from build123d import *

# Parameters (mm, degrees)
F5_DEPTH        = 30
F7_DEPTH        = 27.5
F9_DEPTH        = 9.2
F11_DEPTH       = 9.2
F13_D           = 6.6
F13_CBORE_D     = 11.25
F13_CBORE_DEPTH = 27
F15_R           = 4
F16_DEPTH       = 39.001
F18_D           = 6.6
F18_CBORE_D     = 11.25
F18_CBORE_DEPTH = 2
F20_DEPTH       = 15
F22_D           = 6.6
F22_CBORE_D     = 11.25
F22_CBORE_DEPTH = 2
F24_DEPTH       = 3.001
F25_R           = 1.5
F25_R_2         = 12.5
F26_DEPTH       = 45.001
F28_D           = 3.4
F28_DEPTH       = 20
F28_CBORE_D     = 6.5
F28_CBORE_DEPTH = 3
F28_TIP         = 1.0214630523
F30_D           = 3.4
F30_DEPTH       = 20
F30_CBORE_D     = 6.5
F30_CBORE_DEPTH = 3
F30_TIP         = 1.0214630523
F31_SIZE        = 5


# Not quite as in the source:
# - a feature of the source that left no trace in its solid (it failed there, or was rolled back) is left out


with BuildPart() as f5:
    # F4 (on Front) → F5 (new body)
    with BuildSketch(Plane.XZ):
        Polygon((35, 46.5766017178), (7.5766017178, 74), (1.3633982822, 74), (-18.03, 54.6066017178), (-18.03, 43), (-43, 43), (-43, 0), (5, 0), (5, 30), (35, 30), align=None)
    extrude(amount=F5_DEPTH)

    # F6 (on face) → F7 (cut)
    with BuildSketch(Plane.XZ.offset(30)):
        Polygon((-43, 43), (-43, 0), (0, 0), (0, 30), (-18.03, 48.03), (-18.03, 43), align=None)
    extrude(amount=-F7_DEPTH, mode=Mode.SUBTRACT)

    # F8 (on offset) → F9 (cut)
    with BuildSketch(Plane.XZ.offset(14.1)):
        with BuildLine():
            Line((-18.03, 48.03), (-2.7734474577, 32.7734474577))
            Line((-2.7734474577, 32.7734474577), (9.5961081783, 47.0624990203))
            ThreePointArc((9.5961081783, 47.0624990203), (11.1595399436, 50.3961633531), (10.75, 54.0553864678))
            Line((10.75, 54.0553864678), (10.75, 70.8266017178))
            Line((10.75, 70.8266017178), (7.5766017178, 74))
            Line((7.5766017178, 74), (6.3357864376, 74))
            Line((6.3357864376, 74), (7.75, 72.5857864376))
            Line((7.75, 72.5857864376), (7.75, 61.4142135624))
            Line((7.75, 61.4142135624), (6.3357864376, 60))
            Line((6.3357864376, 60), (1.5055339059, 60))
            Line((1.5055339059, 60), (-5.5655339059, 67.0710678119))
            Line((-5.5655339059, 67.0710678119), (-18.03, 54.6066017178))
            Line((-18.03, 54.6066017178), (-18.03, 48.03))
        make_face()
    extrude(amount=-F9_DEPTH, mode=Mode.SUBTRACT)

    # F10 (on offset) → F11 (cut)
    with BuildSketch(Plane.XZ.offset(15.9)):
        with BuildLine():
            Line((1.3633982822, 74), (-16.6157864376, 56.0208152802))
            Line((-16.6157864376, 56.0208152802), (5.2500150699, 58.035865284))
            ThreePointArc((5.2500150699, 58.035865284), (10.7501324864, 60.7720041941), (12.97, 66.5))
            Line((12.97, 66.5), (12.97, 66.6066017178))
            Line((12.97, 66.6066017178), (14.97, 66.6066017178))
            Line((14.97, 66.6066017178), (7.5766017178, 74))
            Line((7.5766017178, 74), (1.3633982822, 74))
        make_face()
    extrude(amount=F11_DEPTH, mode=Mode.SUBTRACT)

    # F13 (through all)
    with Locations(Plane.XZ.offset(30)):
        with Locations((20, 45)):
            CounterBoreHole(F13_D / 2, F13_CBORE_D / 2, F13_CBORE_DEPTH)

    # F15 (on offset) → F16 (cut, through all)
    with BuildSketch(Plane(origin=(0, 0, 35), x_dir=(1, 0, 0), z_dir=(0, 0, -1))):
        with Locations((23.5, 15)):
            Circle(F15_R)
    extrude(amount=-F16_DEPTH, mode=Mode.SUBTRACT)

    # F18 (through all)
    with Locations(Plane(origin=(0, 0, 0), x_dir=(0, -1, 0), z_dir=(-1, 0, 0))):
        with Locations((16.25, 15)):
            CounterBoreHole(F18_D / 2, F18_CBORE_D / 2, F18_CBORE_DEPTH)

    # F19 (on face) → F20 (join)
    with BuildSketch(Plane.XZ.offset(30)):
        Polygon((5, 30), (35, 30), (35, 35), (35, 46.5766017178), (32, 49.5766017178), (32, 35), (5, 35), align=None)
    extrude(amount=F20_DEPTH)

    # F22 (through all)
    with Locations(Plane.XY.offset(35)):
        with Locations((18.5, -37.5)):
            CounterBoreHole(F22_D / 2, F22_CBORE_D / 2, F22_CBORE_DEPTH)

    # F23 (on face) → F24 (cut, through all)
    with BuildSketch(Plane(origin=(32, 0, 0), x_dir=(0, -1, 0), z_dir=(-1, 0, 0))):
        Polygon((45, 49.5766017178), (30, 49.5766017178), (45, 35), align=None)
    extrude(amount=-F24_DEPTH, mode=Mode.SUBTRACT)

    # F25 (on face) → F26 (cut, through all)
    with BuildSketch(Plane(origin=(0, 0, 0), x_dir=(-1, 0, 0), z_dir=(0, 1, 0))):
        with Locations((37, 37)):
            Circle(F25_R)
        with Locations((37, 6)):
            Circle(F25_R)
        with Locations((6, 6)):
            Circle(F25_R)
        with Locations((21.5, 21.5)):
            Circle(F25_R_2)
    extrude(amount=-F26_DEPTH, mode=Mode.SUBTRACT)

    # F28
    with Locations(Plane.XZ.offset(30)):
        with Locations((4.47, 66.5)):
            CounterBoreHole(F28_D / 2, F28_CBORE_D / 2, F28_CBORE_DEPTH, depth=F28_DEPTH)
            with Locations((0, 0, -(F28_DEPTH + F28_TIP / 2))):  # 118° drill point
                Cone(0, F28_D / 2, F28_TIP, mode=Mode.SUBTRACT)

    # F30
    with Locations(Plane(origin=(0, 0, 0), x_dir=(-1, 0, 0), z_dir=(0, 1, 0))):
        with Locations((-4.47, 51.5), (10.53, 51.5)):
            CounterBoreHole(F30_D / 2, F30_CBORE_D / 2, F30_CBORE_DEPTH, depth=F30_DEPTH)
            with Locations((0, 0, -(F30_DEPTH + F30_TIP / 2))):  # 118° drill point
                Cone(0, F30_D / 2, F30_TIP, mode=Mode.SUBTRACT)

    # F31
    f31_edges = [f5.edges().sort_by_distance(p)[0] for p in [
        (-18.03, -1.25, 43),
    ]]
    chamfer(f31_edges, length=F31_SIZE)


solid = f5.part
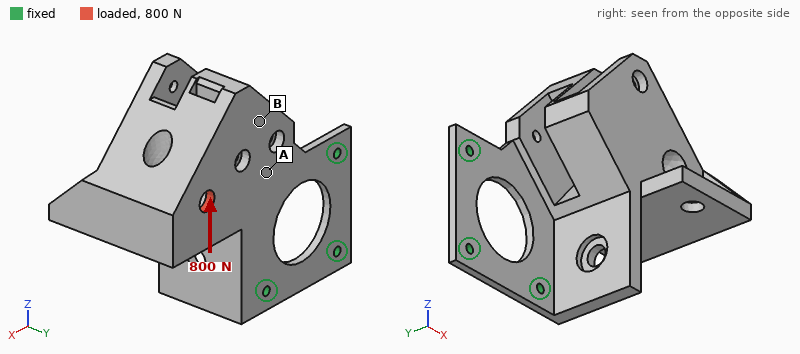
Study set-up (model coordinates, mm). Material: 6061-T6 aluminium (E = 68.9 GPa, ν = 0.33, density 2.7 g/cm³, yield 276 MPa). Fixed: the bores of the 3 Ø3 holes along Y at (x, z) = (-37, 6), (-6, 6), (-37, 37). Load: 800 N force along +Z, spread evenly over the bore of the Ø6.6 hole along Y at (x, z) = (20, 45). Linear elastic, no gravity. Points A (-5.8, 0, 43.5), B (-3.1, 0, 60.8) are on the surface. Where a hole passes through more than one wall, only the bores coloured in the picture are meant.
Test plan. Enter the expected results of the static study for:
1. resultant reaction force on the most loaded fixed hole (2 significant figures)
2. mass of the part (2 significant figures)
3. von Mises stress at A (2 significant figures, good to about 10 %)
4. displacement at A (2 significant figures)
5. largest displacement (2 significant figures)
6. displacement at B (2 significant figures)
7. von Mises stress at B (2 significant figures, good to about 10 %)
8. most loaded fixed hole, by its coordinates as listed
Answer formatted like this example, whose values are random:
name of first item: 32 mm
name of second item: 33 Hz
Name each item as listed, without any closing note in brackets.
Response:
resultant reaction force on the most loaded fixed hole: 1.1 kN
mass of the part: 120 g
von Mises stress at A: 13 MPa
displacement at A: 13 µm
largest displacement: 55 µm
displacement at B: 34 µm
von Mises stress at B: 4.9 MPa
most loaded fixed hole, by its coordinates as listed: (-6, 6)
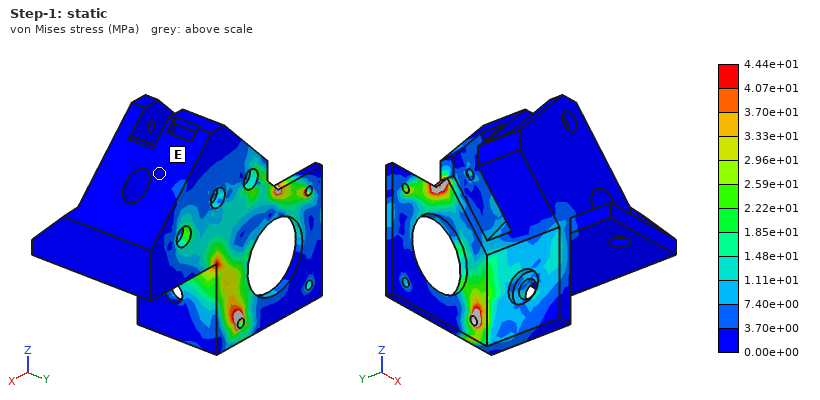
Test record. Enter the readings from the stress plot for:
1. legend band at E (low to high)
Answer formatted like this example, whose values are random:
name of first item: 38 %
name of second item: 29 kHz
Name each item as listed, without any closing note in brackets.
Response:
legend band at E: 0.00e+00 to 3.70e+00 MPa
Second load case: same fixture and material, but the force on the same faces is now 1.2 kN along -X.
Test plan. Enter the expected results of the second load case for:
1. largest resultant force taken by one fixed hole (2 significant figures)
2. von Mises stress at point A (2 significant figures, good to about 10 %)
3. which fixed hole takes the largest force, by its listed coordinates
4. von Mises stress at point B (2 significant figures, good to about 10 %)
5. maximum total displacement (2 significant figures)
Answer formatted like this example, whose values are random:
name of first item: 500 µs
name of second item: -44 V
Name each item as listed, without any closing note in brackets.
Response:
largest resultant force taken by one fixed hole: 1.2 kN
von Mises stress at point A: 26 MPa
which fixed hole takes the largest force, by its listed coordinates: (-37, 37)
von Mises stress at point B: 8.1 MPa
maximum total displacement: 76 µm
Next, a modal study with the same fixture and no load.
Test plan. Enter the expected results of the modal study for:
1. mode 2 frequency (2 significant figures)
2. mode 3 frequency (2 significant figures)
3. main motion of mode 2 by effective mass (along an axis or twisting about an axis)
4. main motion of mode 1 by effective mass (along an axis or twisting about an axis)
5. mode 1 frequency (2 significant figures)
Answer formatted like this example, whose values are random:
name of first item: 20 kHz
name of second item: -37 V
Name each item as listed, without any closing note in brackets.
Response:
mode 2 frequency: 680 Hz
mode 3 frequency: 2600 Hz
main motion of mode 2 by effective mass: along X
main motion of mode 1 by effective mass: along Y
mode 1 frequency: 210 Hz
